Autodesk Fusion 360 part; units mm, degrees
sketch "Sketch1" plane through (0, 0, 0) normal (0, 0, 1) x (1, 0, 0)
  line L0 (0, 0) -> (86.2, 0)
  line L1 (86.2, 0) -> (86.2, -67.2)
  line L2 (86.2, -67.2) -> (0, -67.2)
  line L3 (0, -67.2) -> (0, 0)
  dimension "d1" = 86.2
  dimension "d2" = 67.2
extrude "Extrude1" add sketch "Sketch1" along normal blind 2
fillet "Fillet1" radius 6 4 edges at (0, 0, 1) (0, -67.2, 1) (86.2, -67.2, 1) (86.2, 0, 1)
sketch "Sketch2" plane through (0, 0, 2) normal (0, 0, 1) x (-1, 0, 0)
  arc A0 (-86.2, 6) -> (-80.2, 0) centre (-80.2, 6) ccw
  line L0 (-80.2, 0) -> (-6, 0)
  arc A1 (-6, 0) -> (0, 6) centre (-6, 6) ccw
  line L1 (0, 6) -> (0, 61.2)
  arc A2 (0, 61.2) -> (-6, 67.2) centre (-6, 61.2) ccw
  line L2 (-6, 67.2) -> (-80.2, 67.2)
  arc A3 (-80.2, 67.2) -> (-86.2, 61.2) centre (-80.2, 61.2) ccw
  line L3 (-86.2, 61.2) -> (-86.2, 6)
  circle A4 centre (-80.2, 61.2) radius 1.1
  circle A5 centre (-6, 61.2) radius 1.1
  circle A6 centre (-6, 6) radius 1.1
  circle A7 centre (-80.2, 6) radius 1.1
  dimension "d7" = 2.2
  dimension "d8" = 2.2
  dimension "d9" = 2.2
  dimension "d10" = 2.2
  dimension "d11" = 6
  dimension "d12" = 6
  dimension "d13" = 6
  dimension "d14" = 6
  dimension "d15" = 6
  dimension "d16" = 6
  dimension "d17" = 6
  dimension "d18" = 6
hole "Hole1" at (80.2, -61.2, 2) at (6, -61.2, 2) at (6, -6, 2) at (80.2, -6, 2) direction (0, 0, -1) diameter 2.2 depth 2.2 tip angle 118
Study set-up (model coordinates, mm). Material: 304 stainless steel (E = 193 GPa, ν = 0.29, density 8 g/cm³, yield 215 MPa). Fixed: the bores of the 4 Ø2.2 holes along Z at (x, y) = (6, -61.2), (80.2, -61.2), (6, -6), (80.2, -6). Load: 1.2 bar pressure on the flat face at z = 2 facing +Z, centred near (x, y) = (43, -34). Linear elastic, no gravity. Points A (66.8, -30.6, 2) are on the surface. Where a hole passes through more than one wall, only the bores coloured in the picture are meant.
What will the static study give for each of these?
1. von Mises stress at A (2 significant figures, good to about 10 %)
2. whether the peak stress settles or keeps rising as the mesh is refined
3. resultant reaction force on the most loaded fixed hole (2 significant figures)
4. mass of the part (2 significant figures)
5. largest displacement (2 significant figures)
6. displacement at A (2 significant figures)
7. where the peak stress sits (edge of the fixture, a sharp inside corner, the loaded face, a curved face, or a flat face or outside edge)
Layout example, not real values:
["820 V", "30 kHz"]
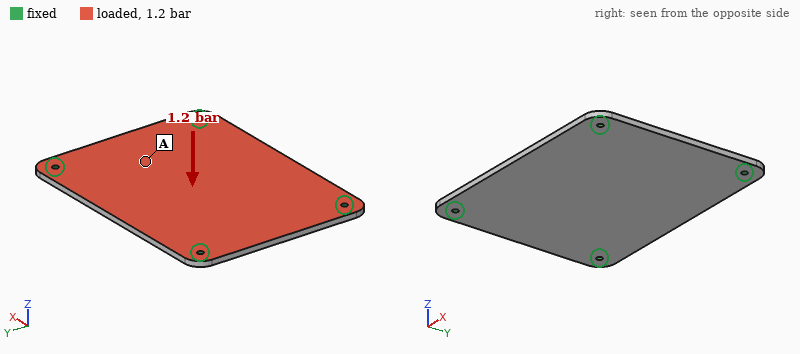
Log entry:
["31 MPa", "keeps rising", "170 N", "92 g", "0.14 mm", "0.085 mm", "edge of the fixture"]
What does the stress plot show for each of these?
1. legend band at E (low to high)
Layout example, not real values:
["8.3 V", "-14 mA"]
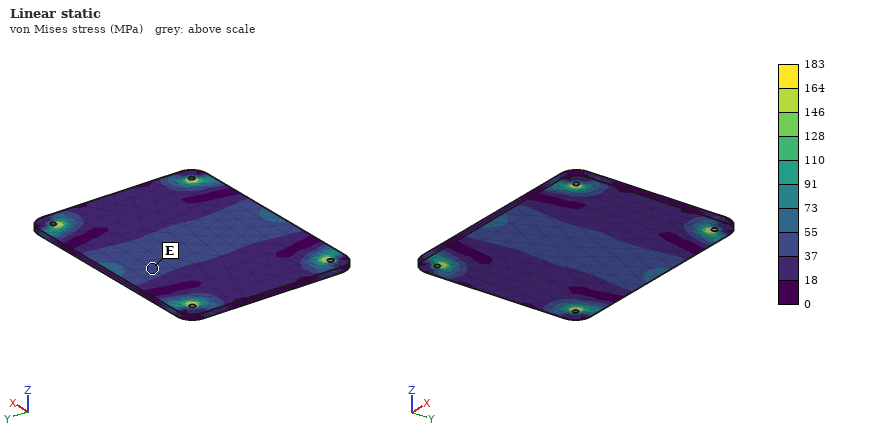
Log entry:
["37 to 55 MPa"]
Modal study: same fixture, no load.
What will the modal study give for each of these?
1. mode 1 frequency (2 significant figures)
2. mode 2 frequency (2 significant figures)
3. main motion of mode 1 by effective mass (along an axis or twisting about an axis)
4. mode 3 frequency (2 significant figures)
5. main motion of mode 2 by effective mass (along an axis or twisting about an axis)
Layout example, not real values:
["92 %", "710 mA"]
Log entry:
["1400 Hz", "2200 Hz", "along Z", "3100 Hz", "twisting about X"]
